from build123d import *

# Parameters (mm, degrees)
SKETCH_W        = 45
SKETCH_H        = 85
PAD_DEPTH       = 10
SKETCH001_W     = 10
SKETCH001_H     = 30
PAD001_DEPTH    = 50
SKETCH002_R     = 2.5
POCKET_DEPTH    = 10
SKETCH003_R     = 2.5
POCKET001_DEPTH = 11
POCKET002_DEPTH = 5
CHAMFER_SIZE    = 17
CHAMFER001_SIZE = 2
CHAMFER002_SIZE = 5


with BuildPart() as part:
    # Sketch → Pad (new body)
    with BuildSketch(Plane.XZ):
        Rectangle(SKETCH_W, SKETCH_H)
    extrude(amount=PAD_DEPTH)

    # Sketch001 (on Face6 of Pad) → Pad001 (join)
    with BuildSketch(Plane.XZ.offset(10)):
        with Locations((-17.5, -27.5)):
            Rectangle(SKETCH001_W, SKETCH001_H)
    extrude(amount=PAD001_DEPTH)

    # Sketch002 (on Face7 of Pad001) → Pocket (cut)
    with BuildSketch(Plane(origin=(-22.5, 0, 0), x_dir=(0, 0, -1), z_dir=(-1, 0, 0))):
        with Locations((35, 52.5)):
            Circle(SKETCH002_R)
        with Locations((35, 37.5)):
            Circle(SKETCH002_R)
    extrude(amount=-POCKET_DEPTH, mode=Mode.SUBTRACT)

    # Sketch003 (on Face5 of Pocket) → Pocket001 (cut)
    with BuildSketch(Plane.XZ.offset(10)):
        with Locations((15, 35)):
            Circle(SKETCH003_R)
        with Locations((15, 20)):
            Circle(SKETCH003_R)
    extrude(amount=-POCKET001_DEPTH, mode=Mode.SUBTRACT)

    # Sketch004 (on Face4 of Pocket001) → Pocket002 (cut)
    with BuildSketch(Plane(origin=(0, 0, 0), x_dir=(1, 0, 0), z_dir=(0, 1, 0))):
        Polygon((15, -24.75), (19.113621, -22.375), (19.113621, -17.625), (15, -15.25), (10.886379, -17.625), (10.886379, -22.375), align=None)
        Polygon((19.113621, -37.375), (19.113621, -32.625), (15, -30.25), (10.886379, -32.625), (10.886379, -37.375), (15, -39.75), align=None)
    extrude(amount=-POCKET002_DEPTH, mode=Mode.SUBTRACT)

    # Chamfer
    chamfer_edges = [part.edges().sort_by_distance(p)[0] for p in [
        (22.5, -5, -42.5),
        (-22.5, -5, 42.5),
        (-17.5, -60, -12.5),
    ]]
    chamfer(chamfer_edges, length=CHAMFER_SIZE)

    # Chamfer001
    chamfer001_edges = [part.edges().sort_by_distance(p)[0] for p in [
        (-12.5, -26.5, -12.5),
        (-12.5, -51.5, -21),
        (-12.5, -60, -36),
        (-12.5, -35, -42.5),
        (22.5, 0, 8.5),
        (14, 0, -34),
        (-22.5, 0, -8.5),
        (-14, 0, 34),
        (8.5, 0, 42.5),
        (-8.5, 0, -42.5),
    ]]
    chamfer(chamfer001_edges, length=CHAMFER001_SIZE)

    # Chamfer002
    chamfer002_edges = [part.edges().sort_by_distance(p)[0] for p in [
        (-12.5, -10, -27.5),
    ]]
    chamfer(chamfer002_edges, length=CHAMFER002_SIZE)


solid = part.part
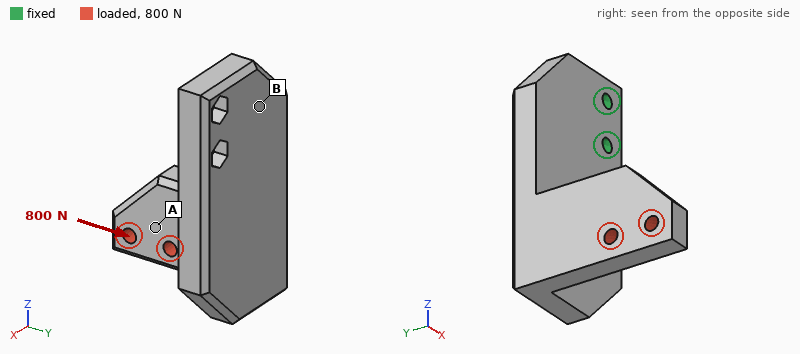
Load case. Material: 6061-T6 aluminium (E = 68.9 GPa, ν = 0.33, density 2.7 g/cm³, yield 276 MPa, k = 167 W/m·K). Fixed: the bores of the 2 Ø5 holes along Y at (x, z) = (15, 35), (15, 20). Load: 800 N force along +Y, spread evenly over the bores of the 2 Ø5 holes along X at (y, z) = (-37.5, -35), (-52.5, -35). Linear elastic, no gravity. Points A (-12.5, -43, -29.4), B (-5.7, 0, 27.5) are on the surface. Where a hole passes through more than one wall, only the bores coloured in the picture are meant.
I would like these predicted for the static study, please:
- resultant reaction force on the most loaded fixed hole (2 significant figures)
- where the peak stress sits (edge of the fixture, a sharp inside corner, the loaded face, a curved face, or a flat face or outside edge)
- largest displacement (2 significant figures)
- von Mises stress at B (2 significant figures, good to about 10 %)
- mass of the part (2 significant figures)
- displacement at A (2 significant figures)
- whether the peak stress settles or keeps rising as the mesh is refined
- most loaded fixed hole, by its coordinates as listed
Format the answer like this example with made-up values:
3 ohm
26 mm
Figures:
2.9 kN
edge of the fixture
0.77 mm
50 MPa
130 g
0.55 mm
keeps rising
(15, 20)
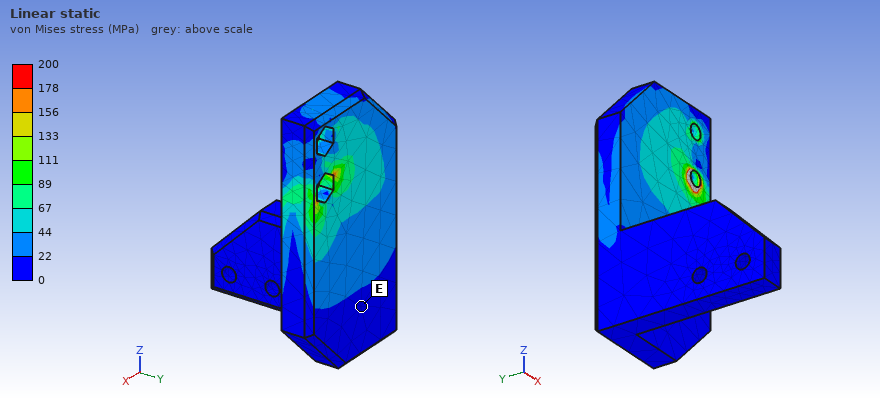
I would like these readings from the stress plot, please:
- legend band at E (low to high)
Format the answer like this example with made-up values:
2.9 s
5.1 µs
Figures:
0 to 22 MPa
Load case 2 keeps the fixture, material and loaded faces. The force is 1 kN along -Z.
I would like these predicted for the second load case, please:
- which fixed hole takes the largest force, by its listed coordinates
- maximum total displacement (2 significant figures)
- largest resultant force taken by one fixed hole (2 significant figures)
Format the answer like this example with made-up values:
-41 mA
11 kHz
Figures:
(15, 20)
0.76 mm
2.6 kN
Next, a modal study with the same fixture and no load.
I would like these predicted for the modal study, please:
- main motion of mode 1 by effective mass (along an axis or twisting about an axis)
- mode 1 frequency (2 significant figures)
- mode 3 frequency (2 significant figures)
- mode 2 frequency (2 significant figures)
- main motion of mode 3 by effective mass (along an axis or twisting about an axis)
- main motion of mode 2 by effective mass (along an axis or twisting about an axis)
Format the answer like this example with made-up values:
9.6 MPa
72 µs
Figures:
along Y
830 Hz
2900 Hz
1400 Hz
along X
along X
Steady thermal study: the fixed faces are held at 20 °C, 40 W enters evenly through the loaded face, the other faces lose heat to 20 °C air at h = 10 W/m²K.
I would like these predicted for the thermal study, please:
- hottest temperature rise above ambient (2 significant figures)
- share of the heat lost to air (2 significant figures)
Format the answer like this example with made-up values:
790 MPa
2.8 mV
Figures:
69 K
8.7 %
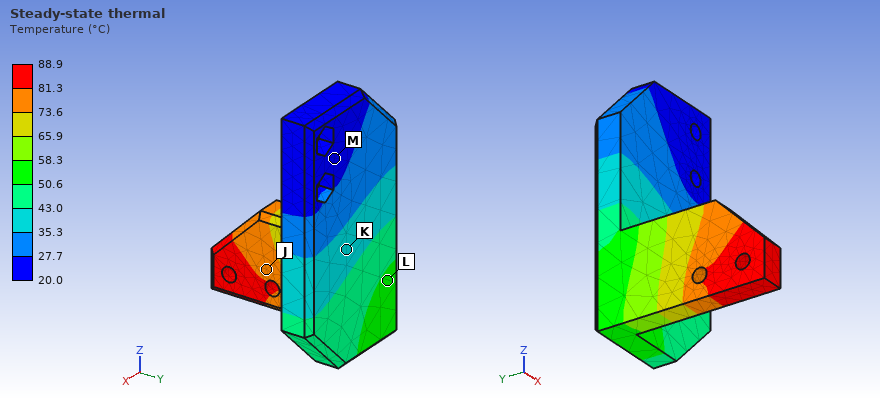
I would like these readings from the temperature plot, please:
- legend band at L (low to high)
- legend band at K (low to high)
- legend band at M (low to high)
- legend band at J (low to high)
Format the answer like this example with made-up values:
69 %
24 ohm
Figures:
50.6 to 58.3 °C
35.3 to 43.0 °C
20.0 to 27.7 °C
73.6 to 81.3 °C
